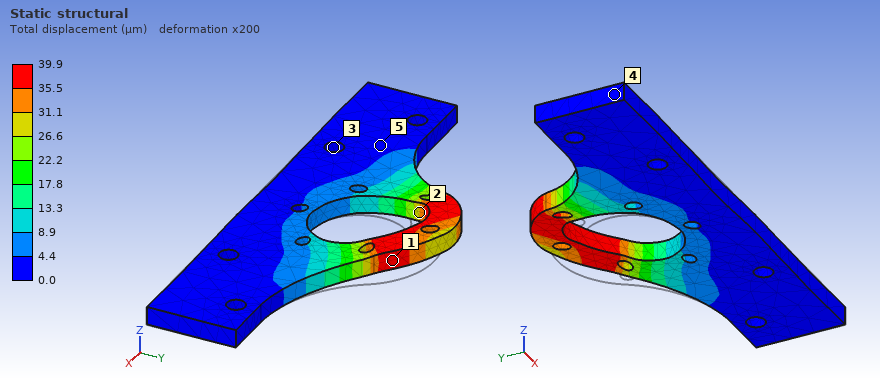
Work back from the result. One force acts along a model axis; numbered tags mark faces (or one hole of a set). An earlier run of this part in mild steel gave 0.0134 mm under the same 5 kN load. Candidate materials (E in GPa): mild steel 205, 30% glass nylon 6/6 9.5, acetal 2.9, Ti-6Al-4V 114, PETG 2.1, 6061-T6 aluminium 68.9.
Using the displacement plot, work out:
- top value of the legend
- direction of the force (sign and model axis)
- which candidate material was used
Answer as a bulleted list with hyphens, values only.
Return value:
- 39.9 µm
- -X
- 6061-T6 aluminium
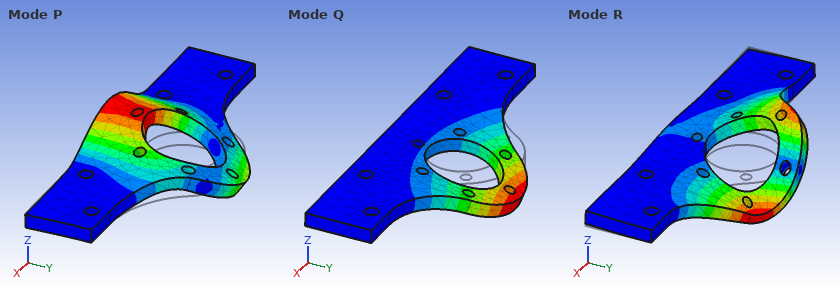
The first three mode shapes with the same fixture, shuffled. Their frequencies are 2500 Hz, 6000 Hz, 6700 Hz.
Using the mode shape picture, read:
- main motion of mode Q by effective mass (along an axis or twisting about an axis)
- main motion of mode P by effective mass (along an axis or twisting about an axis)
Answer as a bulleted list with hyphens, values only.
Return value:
- along Z
- along Z
